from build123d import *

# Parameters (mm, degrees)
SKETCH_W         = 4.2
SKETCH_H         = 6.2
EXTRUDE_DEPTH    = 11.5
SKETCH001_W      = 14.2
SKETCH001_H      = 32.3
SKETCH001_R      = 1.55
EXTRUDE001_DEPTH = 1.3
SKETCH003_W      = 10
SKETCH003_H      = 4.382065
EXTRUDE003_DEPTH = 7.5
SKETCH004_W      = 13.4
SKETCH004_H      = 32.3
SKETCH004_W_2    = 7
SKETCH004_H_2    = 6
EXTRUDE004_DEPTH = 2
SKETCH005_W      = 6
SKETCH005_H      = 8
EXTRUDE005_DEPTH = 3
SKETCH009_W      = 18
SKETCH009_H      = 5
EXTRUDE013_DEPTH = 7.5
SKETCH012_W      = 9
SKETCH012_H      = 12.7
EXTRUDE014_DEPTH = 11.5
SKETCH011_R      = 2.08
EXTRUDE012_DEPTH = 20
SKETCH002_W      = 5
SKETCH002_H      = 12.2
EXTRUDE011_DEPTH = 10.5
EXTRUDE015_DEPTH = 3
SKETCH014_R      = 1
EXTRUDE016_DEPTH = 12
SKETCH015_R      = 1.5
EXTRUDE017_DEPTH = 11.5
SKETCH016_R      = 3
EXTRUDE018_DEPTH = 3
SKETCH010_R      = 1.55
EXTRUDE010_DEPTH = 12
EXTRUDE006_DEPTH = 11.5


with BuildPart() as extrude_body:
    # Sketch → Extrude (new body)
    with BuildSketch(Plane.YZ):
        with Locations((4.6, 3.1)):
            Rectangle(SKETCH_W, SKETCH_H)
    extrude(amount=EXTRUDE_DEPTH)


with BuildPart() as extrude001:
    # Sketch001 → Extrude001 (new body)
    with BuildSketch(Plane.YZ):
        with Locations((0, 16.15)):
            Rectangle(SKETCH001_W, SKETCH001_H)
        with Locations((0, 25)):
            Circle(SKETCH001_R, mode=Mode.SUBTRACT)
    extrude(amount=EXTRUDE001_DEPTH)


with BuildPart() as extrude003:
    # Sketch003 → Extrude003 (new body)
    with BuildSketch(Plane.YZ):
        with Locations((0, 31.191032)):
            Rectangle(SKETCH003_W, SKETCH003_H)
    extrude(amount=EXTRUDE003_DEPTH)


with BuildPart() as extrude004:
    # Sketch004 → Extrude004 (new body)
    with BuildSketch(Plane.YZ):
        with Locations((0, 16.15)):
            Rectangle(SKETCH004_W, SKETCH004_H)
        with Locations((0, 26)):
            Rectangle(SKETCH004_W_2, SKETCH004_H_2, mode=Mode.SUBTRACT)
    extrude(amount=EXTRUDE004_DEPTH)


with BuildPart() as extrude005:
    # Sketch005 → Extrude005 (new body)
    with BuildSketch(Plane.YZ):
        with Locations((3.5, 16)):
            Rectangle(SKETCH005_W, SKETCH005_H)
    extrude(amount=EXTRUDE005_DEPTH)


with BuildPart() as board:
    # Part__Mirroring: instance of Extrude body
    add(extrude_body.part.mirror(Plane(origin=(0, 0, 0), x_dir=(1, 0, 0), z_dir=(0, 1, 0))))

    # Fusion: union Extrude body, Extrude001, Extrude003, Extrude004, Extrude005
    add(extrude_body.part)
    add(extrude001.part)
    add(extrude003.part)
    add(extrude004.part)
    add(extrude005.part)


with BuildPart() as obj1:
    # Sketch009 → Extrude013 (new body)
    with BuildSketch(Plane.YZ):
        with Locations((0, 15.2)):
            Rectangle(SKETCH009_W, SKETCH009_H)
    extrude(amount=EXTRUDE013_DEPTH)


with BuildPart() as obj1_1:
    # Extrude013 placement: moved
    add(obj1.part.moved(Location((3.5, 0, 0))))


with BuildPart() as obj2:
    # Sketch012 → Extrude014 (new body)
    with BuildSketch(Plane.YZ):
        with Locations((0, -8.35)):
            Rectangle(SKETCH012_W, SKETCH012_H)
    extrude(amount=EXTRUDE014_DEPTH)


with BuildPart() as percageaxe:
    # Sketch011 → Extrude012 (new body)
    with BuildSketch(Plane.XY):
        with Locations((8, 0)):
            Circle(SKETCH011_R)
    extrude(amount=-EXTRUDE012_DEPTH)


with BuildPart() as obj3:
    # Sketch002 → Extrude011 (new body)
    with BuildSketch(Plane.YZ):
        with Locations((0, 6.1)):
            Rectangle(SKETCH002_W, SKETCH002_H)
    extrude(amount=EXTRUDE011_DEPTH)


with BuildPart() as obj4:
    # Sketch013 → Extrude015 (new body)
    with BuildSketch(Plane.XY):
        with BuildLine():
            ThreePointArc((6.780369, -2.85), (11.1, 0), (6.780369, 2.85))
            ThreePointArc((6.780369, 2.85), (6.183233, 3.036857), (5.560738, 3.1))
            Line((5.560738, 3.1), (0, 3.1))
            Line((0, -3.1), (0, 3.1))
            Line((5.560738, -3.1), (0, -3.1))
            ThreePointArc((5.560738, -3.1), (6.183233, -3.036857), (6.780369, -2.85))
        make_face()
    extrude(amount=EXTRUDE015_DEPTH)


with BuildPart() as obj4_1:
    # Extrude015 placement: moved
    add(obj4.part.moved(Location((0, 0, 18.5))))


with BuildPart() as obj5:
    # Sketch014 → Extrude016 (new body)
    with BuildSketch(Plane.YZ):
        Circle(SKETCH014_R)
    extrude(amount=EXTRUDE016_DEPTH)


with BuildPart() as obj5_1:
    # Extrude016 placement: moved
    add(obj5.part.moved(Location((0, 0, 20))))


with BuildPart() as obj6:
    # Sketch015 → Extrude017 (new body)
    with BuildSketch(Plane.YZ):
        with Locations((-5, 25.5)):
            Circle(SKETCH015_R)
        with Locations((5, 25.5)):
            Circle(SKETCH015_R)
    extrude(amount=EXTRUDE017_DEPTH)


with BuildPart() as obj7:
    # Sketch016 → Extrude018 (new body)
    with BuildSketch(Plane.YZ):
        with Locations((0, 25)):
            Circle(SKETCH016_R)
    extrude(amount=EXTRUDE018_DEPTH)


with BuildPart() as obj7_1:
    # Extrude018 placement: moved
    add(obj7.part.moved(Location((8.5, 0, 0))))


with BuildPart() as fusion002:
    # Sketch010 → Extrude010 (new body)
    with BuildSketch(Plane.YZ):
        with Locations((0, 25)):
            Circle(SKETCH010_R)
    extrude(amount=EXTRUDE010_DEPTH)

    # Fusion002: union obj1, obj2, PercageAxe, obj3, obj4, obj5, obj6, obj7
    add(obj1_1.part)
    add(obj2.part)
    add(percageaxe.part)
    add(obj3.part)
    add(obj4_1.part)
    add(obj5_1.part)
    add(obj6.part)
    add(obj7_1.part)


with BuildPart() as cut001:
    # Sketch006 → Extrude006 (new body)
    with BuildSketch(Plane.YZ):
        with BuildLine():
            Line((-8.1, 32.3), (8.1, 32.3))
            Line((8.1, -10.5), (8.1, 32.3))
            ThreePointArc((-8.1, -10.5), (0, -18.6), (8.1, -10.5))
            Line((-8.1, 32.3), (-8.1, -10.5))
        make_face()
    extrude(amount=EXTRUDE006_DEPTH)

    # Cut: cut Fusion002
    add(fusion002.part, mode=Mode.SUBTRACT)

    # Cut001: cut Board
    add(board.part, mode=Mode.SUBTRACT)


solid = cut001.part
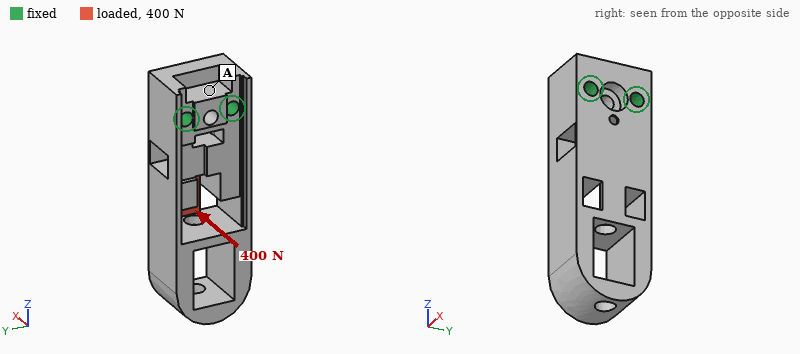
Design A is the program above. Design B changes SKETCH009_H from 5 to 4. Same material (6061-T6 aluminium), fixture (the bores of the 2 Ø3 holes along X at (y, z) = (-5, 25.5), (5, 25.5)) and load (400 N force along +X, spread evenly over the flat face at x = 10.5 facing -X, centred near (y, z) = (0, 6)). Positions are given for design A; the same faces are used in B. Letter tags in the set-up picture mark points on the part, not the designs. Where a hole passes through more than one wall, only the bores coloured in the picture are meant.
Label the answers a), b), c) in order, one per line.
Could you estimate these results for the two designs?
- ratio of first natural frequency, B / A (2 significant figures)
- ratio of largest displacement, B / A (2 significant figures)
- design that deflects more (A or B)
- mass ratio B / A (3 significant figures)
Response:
a) 1.0
b) 0.88
c) A
d) 1.03
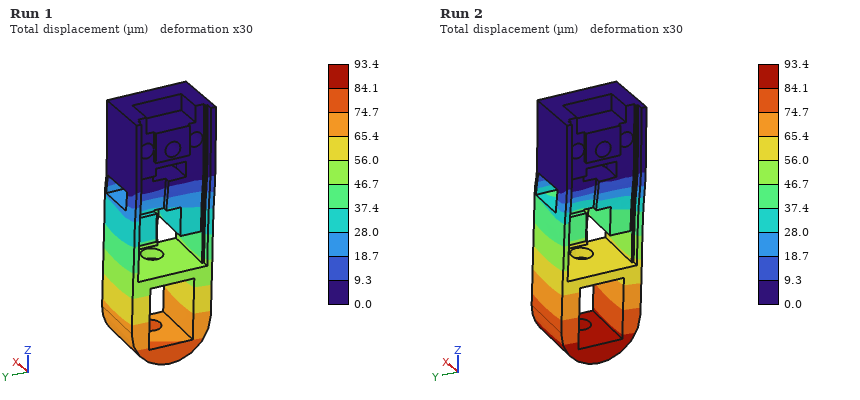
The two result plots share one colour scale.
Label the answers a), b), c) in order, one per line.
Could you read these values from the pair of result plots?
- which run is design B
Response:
a) Run 1
